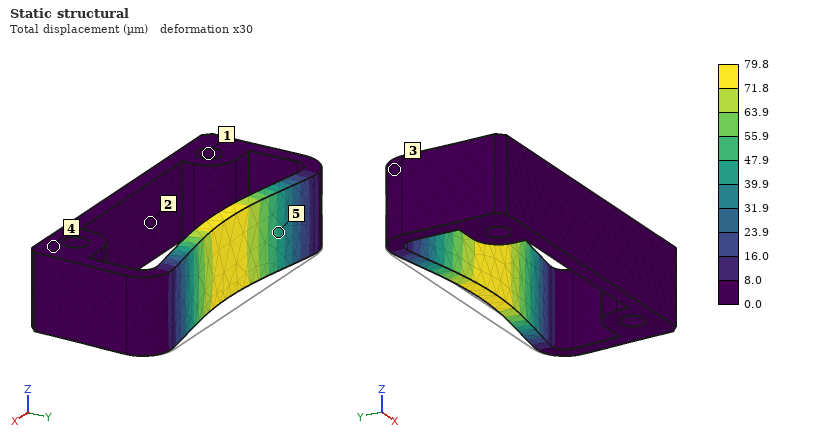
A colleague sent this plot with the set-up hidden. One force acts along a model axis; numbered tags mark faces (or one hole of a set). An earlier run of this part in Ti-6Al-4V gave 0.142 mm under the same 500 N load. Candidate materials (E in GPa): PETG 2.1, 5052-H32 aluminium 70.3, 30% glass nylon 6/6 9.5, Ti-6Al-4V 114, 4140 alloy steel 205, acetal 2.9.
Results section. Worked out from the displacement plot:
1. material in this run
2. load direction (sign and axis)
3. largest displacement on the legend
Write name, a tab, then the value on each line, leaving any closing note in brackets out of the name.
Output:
material in this run	4140 alloy steel
load direction	-Y
largest displacement on the legend	79.8 µm
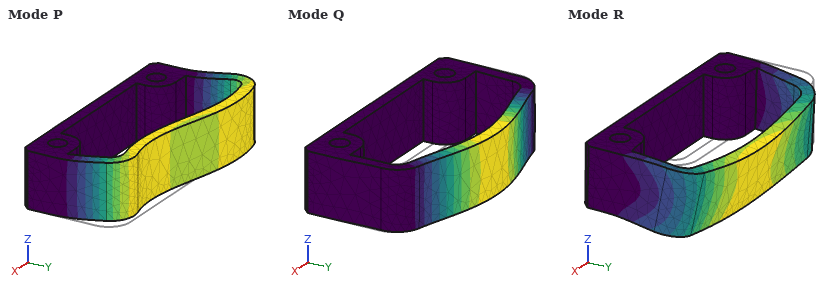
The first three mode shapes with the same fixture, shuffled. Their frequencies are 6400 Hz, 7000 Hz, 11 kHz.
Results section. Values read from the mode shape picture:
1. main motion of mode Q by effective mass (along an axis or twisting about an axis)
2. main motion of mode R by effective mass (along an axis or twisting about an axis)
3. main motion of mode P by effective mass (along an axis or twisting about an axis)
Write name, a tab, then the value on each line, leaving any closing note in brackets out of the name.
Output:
main motion of mode Q by effective mass	along Y
main motion of mode R by effective mass	along Z
main motion of mode P by effective mass	along X
